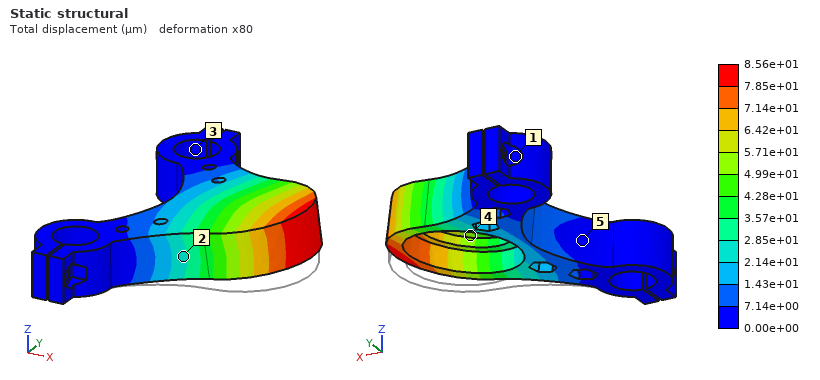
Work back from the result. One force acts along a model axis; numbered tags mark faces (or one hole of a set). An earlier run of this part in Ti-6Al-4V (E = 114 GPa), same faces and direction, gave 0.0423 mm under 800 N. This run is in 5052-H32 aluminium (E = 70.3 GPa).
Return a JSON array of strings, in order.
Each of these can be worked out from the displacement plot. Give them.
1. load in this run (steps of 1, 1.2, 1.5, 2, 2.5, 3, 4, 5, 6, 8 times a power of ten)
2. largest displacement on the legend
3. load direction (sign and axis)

["1 kN", "8.56e+01 µm", "+Z"]
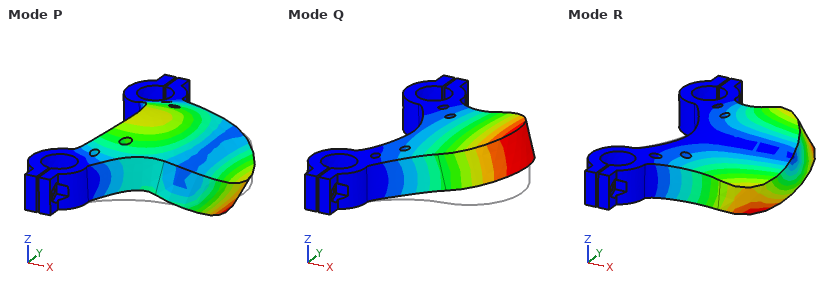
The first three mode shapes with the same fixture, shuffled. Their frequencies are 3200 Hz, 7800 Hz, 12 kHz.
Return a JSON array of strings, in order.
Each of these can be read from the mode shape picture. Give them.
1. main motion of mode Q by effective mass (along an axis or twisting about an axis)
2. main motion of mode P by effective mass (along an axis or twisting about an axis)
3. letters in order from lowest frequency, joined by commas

["along Z", "along Z", "Q, R, P"]
